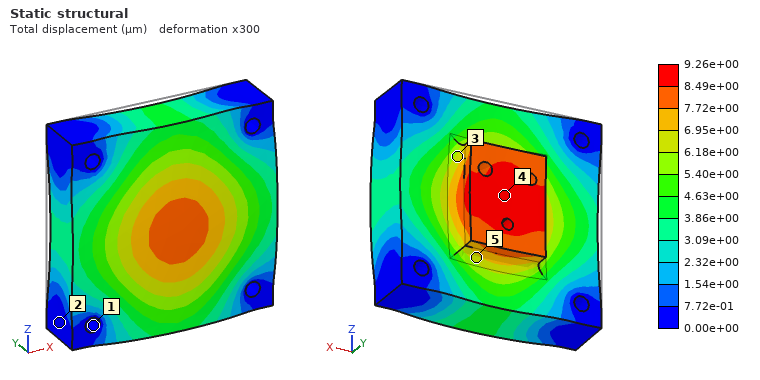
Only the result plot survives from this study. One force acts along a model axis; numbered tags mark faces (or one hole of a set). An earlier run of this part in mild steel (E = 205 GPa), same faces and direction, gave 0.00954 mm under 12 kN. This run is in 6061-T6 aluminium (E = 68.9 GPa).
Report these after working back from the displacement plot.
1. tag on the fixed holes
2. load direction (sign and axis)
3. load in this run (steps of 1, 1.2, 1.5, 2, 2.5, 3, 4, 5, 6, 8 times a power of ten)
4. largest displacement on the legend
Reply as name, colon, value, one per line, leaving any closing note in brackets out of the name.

tag on the fixed holes: 1
load direction: -Y
load in this run: 4 kN
largest displacement on the legend: 9.26e+00 µm
